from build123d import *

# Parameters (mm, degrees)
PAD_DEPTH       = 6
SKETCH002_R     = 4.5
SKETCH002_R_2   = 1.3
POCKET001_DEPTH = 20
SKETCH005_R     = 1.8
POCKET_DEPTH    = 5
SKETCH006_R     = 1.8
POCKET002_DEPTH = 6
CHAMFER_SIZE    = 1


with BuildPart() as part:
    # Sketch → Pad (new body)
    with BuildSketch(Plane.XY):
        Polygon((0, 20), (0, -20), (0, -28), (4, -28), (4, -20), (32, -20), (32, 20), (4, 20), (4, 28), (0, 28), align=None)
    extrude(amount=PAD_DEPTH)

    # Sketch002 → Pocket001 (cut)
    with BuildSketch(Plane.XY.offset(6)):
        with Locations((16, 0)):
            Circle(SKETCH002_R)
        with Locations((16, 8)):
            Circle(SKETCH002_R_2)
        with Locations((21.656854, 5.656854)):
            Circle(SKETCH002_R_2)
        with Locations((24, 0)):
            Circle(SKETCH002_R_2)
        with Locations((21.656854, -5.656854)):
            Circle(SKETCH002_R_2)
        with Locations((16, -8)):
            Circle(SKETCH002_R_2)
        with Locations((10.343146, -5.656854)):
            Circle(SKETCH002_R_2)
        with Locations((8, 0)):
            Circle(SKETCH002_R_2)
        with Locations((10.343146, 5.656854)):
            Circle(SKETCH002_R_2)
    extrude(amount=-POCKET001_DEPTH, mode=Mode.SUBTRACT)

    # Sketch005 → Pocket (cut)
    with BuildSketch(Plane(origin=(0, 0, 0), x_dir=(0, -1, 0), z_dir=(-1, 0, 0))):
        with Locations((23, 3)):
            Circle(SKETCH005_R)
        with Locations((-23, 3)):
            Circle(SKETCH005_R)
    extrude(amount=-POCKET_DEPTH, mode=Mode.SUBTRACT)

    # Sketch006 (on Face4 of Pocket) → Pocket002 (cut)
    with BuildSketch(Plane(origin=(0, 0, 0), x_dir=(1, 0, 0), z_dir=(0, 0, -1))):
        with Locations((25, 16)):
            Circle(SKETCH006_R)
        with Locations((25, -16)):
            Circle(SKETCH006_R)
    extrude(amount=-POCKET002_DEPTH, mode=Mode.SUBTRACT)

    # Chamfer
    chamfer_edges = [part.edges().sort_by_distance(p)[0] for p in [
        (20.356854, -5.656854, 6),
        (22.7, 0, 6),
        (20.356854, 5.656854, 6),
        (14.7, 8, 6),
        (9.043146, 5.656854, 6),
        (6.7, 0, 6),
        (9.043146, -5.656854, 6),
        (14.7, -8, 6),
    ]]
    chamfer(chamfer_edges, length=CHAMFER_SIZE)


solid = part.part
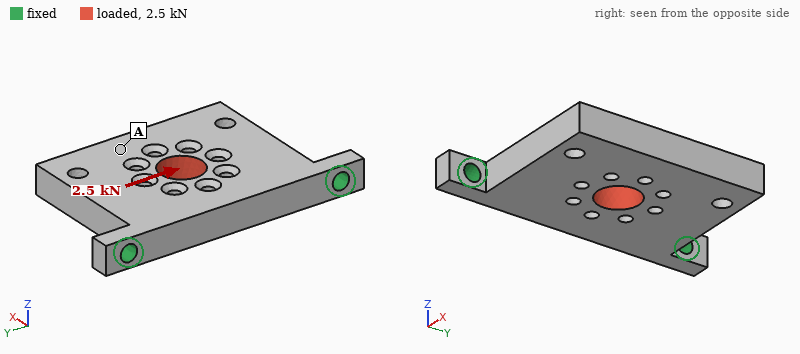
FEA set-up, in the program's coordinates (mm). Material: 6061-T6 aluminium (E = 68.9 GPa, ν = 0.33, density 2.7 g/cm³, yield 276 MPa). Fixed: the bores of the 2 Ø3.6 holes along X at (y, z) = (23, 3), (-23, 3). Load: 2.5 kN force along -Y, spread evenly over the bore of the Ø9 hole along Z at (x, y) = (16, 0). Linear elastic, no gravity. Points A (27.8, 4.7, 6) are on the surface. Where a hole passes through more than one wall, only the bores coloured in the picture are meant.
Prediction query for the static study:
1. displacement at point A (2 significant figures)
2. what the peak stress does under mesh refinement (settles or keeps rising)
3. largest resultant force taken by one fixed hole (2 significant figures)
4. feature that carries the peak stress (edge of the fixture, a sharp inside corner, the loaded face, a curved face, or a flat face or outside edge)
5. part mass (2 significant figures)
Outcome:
21 µm
keeps rising
1.5 kN
edge of the fixture
19 g
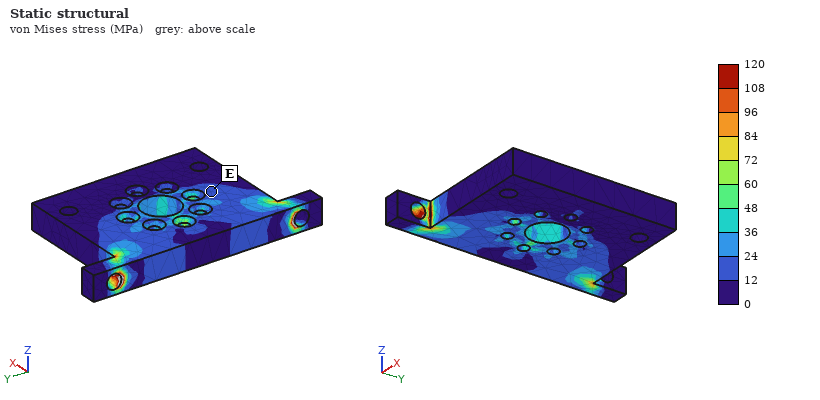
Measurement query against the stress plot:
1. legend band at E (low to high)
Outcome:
12 to 24 MPa
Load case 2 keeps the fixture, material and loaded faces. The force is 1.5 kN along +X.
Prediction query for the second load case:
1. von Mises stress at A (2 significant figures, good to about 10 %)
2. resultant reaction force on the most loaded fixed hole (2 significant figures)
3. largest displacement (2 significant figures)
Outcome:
9.1 MPa
870 N
13 µm
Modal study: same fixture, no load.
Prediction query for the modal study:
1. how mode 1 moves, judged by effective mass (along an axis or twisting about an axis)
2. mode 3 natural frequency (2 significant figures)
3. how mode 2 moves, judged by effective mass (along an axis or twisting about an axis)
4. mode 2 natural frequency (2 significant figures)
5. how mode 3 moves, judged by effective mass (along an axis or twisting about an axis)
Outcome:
along Z
12 kHz
twisting about X
7500 Hz
along Z
